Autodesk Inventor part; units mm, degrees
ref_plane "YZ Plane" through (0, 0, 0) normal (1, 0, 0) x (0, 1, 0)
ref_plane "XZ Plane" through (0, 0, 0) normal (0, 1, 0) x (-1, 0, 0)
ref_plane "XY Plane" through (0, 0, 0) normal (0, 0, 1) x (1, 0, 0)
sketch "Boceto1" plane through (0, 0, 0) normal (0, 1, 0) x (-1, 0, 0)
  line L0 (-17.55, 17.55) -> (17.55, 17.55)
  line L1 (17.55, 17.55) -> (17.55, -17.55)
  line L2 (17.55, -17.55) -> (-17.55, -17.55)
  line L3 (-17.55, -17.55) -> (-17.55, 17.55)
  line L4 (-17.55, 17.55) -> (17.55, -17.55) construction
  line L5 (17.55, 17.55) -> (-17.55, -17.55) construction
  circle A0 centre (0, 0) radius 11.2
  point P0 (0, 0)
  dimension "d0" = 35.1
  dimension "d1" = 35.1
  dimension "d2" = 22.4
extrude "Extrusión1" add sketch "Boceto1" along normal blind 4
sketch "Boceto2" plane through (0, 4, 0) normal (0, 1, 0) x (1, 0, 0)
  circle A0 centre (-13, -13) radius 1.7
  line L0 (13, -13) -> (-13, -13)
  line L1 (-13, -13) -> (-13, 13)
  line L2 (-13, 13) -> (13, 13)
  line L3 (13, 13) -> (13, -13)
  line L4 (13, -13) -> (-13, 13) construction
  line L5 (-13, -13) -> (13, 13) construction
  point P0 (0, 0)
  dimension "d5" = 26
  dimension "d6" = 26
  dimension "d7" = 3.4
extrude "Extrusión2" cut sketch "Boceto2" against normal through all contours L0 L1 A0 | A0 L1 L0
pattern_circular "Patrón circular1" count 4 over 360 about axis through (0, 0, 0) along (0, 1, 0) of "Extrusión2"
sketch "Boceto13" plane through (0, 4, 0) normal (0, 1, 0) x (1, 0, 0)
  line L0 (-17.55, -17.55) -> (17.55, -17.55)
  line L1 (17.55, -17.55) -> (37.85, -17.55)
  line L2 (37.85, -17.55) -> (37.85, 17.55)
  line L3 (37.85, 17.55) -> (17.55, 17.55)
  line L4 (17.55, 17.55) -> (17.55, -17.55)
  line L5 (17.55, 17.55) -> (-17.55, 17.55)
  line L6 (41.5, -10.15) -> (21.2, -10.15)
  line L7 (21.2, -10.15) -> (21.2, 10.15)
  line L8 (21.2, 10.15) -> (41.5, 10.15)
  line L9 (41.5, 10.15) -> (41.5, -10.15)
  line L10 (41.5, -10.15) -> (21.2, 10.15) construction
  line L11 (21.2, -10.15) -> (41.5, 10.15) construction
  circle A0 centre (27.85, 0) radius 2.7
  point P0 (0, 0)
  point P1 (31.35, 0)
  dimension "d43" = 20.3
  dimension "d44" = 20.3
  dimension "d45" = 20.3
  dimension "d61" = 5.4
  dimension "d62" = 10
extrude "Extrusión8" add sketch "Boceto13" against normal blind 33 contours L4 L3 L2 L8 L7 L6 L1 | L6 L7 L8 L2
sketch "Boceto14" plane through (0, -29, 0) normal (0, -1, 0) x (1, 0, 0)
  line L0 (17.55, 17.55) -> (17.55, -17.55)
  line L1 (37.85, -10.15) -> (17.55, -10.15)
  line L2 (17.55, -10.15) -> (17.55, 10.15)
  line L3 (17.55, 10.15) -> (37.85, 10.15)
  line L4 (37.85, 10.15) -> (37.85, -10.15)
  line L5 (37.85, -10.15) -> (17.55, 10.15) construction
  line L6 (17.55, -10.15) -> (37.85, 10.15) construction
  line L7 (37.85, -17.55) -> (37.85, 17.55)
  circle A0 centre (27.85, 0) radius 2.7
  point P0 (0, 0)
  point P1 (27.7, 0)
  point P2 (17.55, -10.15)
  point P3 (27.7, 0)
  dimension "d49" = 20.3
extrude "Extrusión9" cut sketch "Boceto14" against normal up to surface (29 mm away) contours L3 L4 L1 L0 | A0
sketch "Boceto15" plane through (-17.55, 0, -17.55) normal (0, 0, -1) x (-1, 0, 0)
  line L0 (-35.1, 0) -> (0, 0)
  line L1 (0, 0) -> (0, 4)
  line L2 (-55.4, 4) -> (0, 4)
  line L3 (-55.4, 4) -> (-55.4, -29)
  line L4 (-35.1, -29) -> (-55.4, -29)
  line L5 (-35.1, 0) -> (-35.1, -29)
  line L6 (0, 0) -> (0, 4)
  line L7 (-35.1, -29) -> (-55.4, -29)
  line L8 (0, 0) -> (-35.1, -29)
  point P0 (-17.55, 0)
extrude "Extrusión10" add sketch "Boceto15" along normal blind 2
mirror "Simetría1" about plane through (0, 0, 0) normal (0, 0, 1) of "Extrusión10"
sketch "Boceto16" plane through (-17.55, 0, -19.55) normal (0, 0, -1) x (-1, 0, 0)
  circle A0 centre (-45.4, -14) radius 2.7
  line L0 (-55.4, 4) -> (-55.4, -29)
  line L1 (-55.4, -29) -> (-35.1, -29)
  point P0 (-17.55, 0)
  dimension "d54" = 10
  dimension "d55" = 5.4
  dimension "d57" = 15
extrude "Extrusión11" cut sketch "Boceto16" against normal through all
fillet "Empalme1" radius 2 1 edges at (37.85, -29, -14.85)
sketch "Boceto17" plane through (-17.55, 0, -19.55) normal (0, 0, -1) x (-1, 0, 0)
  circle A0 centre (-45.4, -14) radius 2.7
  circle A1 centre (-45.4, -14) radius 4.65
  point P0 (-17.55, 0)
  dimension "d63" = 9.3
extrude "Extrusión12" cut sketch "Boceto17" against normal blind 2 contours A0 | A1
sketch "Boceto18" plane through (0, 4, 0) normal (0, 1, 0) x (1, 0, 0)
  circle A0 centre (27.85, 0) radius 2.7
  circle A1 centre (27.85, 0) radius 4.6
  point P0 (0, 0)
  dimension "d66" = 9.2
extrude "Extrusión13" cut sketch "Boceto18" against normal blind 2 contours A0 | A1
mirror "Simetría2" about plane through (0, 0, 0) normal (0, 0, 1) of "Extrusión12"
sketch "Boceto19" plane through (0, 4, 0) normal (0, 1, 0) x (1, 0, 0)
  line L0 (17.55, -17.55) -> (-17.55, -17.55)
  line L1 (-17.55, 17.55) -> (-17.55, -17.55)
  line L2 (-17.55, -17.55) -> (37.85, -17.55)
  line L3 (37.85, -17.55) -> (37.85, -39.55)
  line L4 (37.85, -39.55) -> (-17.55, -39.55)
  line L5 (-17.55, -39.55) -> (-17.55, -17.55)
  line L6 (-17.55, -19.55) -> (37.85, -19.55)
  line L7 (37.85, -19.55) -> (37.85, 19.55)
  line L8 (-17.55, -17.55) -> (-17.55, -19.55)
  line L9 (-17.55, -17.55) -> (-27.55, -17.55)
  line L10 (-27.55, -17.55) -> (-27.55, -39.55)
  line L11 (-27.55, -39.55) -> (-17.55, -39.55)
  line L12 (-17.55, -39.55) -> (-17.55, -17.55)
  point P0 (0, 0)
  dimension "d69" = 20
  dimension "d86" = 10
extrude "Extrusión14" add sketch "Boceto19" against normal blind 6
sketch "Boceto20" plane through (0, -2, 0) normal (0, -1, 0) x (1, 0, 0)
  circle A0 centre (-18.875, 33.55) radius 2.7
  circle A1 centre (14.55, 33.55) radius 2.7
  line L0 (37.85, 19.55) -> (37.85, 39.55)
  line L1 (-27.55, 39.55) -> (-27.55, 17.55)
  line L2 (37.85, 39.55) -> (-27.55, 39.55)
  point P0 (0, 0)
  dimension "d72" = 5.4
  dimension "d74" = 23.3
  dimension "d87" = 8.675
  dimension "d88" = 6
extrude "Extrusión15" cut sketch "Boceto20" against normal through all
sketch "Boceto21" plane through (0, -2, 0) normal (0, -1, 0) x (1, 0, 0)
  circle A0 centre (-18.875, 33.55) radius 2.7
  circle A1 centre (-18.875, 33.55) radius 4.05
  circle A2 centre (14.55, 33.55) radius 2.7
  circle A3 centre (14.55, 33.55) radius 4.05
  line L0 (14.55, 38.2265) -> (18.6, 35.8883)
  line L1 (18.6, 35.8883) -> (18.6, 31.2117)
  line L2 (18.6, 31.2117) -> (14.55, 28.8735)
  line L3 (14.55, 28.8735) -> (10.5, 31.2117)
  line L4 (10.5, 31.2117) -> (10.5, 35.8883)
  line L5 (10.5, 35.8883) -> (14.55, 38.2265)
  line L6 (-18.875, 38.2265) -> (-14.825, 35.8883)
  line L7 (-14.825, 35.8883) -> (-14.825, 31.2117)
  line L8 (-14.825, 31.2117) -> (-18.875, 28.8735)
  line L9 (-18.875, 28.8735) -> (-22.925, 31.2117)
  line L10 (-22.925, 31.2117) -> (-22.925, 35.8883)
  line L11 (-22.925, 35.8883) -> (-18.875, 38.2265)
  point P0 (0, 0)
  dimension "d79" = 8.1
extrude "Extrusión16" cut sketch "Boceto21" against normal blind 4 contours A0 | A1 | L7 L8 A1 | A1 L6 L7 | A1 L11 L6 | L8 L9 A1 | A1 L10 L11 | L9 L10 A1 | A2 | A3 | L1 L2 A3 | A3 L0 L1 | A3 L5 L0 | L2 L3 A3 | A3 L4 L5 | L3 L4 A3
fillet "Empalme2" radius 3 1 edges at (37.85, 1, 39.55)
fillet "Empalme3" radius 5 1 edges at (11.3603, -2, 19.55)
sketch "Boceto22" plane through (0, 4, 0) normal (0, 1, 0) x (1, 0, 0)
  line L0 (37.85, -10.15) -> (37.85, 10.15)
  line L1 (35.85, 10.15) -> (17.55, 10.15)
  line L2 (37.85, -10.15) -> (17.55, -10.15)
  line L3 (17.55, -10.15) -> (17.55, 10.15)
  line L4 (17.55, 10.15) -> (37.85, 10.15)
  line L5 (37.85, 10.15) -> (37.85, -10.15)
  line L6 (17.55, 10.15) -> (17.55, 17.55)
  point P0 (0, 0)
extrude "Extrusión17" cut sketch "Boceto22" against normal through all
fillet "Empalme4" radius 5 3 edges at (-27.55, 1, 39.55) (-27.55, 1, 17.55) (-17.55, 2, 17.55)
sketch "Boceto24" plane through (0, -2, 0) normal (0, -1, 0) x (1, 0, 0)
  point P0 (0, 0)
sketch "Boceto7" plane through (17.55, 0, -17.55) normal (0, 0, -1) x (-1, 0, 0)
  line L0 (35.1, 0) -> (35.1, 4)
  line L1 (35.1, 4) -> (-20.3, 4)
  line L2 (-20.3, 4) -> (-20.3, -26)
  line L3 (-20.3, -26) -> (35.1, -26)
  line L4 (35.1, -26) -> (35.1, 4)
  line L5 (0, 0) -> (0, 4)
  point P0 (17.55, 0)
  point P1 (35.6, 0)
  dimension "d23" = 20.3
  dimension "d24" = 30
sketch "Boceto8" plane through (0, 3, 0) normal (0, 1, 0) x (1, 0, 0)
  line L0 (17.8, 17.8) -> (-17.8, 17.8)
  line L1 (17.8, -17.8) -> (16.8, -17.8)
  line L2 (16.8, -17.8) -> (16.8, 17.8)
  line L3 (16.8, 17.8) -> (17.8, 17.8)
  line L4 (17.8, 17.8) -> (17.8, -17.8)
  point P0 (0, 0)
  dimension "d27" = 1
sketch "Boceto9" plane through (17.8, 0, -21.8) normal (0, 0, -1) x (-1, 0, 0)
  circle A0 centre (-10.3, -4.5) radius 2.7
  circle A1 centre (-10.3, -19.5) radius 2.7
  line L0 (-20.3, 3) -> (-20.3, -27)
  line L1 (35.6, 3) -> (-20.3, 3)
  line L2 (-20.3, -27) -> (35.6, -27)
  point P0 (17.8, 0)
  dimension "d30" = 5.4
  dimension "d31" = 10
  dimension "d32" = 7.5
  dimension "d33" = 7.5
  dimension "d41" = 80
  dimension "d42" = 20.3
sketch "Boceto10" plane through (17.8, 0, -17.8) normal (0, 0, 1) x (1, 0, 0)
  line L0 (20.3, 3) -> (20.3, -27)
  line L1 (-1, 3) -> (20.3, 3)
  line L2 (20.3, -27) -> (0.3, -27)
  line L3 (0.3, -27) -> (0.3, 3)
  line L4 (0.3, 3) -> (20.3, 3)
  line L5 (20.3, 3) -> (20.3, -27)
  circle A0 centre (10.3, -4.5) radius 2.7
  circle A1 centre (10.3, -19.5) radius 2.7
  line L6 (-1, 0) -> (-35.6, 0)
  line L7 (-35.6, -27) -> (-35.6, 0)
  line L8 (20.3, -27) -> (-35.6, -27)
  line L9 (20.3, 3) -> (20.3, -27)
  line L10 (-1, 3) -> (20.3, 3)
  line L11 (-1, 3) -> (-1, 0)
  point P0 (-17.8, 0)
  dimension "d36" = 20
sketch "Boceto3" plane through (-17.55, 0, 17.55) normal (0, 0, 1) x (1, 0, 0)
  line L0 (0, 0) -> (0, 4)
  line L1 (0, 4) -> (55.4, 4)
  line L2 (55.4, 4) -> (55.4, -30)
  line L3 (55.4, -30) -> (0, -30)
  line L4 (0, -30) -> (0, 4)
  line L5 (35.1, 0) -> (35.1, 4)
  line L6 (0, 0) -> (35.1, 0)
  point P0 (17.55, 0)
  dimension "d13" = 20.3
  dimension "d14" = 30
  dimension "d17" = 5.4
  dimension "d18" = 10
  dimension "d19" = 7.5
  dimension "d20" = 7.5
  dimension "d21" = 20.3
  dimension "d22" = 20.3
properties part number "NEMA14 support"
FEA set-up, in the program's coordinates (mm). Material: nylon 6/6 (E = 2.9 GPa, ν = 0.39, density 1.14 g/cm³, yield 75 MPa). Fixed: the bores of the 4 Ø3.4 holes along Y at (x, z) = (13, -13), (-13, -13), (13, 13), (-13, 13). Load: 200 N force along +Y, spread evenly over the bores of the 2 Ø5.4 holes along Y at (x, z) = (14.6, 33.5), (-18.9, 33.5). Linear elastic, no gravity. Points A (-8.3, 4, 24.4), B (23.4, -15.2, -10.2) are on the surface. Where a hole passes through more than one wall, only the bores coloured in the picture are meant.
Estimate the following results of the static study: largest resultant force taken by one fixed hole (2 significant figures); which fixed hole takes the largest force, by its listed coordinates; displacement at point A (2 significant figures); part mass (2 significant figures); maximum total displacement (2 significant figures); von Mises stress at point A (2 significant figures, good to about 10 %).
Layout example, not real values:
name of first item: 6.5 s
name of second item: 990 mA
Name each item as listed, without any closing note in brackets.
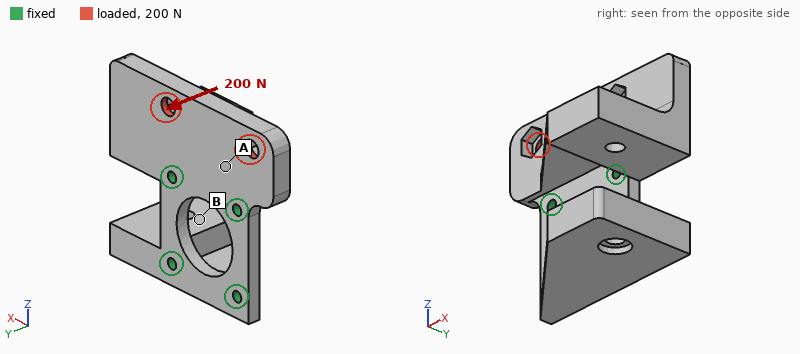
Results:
largest resultant force taken by one fixed hole: 110 N
which fixed hole takes the largest force, by its listed coordinates: (-13, 13)
displacement at point A: 0.35 mm
part mass: 29 g
maximum total displacement: 1.1 mm
von Mises stress at point A: 6.5 MPa
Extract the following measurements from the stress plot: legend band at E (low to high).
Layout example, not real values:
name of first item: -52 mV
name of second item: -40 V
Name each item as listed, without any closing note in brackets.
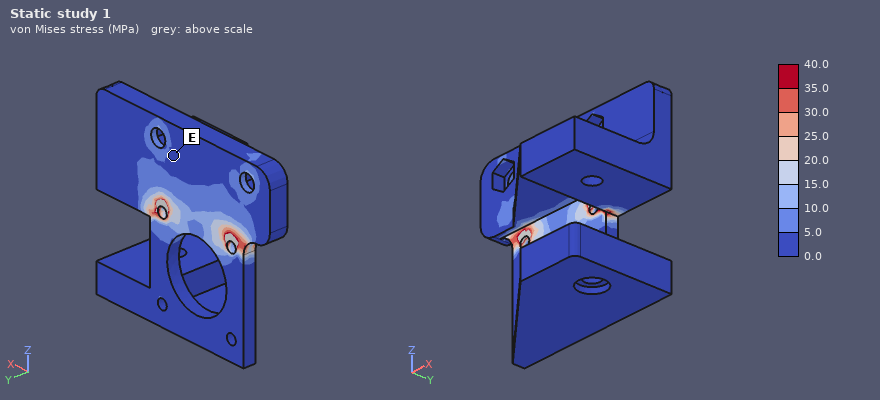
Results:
legend band at E: 0.0 to 5.0 MPa
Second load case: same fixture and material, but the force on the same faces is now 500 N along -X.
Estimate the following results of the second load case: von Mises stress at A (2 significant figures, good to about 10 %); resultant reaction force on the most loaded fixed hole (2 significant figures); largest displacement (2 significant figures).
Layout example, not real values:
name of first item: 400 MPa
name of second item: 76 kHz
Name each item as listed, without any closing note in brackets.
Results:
von Mises stress at A: 9.0 MPa
resultant reaction force on the most loaded fixed hole: 420 N
largest displacement: 0.27 mm
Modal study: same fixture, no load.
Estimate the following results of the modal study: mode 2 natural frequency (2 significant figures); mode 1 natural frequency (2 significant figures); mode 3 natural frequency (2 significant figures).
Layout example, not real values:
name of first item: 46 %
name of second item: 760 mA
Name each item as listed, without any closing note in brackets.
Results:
mode 2 natural frequency: 730 Hz
mode 1 natural frequency: 720 Hz
mode 3 natural frequency: 1400 Hz
